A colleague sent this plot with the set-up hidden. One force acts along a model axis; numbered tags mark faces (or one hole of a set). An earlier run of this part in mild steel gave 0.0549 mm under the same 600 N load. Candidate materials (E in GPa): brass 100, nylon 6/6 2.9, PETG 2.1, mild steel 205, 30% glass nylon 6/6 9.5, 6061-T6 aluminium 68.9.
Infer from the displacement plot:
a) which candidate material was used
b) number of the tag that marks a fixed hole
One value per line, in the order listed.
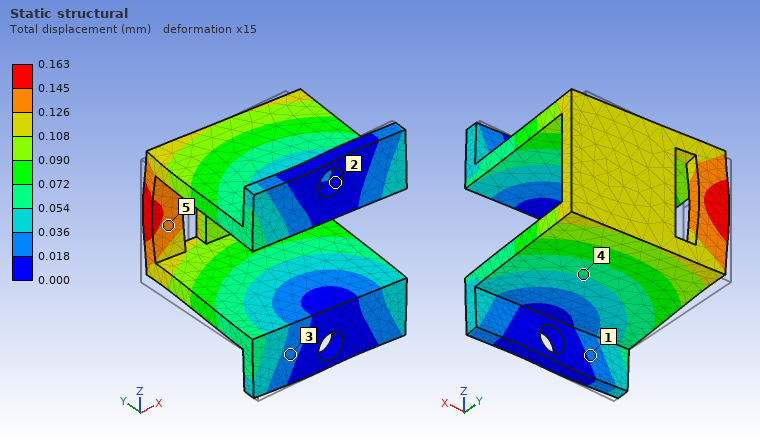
6061-T6 aluminium
2
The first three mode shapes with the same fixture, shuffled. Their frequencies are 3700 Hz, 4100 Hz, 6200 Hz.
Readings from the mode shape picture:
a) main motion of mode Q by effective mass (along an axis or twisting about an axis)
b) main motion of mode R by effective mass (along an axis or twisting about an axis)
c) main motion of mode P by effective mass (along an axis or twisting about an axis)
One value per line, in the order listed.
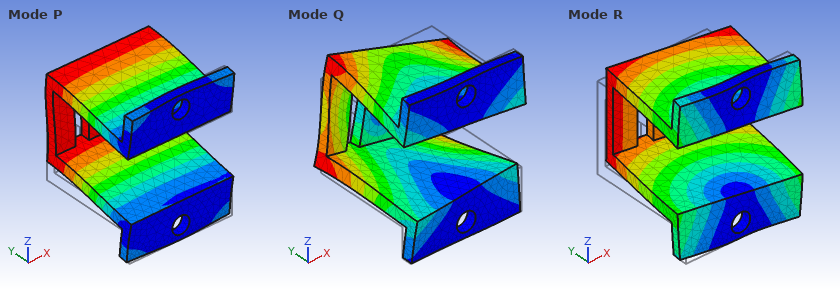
twisting about Y
along X
along Z
